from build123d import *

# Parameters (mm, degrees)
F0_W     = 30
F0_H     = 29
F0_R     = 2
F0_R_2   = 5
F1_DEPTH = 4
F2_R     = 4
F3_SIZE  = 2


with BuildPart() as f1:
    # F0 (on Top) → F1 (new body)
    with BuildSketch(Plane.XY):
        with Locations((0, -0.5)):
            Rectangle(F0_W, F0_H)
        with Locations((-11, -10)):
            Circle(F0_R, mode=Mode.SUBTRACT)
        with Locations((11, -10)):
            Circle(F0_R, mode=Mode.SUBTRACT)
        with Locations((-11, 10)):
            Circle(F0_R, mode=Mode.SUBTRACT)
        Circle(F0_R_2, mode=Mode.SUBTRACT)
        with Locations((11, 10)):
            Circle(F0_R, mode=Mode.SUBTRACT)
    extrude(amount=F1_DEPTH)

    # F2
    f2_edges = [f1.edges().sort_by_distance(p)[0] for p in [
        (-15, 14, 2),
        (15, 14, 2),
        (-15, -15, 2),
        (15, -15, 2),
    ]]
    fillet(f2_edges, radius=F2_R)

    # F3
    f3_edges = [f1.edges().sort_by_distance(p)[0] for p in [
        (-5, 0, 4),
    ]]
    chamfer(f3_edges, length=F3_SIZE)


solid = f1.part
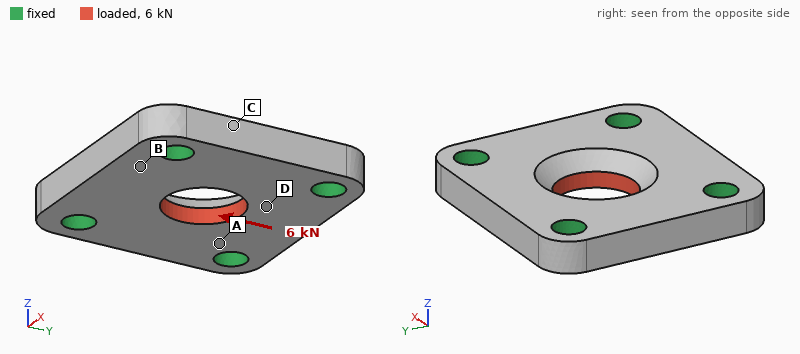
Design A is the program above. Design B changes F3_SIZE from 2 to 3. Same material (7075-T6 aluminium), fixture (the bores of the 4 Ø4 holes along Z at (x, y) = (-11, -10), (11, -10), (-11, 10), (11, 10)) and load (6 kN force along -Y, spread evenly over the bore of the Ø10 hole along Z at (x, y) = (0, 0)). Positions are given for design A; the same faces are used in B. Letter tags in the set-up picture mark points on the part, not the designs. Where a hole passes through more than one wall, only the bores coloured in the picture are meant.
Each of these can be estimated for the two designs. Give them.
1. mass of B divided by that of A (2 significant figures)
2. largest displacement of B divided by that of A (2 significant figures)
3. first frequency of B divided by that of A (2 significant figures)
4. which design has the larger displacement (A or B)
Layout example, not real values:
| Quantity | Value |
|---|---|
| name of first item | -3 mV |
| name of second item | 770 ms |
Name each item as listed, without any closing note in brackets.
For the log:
| Quantity | Value |
|---|---|
| mass of B divided by that of A | 0.97 |
| largest displacement of B divided by that of A | 1.5 |
| first frequency of B divided by that of A | 1.1 |
| which design has the larger displacement | B |
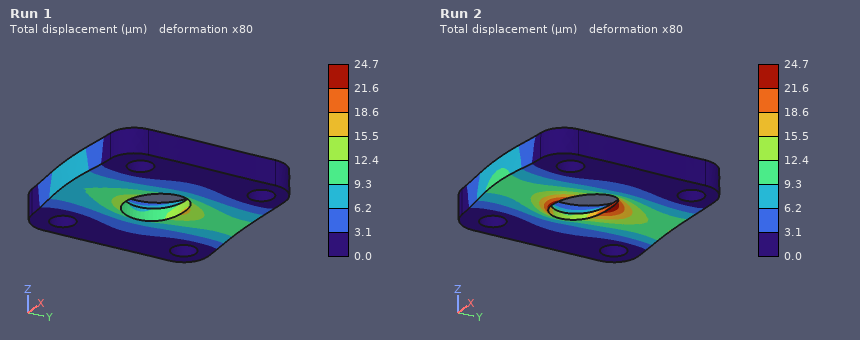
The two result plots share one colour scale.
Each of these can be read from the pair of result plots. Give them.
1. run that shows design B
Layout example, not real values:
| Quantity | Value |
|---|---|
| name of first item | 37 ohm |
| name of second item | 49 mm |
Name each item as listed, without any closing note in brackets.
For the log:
| Quantity | Value |
|---|---|
| run that shows design B | Run 2 |
